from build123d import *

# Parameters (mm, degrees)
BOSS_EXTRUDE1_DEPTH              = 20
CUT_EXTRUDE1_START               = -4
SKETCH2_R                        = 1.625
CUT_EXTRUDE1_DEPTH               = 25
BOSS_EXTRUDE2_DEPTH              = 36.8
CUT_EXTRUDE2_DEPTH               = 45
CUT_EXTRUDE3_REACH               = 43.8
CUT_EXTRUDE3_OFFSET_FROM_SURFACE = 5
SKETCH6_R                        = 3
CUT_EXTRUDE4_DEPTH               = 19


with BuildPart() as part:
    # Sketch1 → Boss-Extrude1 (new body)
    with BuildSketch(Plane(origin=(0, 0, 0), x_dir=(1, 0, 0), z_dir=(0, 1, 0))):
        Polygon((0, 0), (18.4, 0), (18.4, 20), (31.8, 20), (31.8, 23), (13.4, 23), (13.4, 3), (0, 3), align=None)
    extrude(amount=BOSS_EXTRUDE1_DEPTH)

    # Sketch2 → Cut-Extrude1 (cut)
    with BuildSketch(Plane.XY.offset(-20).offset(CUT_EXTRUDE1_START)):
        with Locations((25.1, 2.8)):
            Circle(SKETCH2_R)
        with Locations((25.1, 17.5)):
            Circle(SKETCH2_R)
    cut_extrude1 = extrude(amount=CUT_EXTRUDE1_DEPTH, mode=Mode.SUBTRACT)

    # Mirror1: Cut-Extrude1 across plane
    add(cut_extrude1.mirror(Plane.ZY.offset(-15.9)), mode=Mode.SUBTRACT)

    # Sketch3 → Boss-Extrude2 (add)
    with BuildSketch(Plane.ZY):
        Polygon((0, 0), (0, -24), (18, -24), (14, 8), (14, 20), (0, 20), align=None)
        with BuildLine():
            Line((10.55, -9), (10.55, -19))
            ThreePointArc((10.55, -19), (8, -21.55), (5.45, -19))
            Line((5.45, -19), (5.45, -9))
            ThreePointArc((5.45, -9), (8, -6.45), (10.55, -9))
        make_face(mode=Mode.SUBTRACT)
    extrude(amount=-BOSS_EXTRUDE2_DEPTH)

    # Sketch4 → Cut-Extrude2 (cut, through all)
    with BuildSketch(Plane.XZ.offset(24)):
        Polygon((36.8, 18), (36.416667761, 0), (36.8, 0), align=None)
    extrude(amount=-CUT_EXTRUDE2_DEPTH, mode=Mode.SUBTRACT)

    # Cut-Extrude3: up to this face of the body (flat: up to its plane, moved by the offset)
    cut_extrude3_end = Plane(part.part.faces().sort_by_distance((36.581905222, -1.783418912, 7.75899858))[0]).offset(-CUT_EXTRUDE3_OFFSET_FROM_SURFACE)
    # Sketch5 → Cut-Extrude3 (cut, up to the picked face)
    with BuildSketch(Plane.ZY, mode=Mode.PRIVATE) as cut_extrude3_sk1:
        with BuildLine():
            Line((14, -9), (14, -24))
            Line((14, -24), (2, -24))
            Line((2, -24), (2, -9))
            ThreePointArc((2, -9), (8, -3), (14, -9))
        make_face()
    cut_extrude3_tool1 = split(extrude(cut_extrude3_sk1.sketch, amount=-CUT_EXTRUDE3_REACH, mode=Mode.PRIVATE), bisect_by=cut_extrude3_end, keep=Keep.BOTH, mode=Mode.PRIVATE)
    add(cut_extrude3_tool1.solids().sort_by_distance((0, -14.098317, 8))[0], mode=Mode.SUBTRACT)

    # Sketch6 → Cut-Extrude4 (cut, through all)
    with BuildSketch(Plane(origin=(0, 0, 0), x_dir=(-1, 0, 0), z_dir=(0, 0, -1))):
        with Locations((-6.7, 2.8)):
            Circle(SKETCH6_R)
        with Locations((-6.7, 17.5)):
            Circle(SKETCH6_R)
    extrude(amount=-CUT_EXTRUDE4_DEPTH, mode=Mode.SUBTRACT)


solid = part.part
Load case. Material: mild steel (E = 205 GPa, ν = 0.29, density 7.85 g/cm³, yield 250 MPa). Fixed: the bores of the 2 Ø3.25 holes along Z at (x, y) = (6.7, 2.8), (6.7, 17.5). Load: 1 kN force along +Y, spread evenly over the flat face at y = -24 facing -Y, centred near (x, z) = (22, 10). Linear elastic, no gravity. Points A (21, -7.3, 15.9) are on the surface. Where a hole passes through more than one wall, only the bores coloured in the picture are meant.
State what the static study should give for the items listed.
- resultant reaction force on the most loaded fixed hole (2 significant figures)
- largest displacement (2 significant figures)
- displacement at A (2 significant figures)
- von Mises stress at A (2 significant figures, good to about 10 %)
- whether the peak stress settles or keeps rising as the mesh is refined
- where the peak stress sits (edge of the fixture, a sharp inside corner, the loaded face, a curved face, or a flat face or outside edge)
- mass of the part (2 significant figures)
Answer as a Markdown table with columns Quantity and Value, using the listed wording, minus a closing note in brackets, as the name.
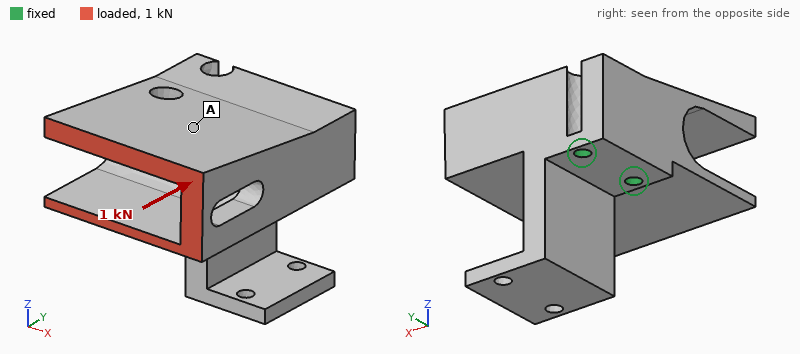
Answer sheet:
| Quantity | Value |
|---|---|
| resultant reaction force on the most loaded fixed hole | 1.3 kN |
| largest displacement | 15 µm |
| displacement at A | 7.6 µm |
| von Mises stress at A | 12 MPa |
| whether the peak stress settles or keeps rising as the mesh is refined | keeps rising |
| where the peak stress sits | edge of the fixture |
| mass of the part | 160 g |
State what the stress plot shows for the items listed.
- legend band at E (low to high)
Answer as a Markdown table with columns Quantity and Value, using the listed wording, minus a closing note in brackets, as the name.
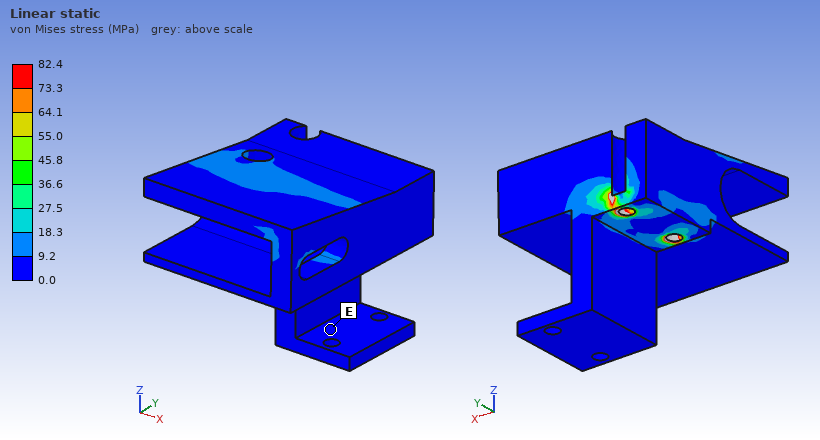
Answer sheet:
| Quantity | Value |
|---|---|
| legend band at E | 0.0 to 9.2 MPa |
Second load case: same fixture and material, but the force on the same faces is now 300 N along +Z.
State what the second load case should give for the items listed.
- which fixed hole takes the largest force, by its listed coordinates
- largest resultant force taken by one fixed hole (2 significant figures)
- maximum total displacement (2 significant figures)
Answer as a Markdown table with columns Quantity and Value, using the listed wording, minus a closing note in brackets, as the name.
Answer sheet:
| Quantity | Value |
|---|---|
| which fixed hole takes the largest force, by its listed coordinates | (6.7, 2.8) |
| largest resultant force taken by one fixed hole | 830 N |
| maximum total displacement | 35 µm |
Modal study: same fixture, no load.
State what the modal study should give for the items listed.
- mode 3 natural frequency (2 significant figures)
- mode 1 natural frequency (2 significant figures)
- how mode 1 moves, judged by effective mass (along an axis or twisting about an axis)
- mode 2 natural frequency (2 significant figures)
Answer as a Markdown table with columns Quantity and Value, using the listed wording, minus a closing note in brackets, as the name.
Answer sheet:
| Quantity | Value |
|---|---|
| mode 3 natural frequency | 5200 Hz |
| mode 1 natural frequency | 2000 Hz |
| how mode 1 moves, judged by effective mass | along Z |
| mode 2 natural frequency | 4600 Hz |
